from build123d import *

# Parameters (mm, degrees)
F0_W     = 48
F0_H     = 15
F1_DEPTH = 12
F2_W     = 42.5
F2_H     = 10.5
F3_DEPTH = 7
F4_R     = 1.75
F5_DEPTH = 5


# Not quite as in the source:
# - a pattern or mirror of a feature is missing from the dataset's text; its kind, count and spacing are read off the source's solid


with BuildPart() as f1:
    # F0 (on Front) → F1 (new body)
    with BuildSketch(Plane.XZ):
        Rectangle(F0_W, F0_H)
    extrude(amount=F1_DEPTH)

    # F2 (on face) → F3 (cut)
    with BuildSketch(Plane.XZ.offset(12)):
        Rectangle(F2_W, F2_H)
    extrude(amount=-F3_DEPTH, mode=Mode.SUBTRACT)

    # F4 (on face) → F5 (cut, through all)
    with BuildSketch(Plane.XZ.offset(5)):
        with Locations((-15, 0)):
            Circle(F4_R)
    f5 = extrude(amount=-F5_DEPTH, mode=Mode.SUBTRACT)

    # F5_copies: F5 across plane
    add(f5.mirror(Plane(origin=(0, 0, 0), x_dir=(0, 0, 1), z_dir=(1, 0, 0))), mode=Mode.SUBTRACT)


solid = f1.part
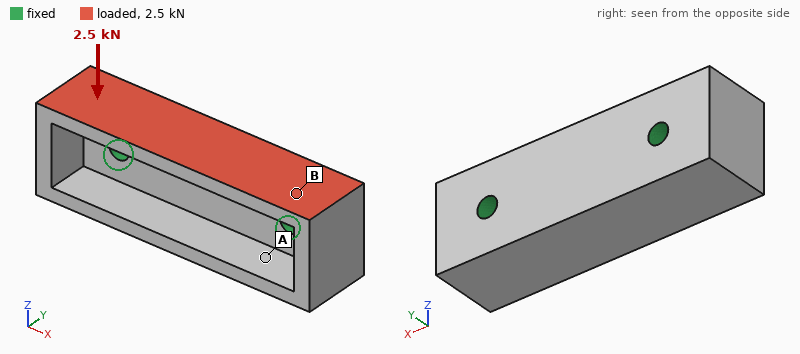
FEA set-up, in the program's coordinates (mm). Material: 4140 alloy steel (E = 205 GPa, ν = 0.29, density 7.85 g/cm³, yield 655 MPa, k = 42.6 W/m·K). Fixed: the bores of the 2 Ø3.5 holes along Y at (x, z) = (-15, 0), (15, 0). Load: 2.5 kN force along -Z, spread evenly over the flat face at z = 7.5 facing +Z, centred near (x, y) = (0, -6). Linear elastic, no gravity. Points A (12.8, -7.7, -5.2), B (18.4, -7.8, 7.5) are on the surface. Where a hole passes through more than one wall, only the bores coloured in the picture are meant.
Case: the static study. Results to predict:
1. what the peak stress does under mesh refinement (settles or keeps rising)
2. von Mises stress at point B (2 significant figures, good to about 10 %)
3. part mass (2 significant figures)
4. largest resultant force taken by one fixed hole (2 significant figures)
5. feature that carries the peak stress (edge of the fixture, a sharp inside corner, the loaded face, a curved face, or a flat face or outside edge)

keeps rising
47 MPa
43 g
1.3 kN
edge of the fixture
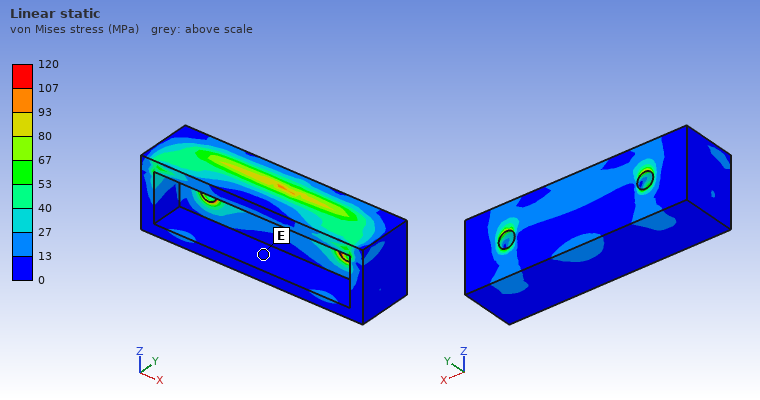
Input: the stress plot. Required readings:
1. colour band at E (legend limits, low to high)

0 to 13 MPa
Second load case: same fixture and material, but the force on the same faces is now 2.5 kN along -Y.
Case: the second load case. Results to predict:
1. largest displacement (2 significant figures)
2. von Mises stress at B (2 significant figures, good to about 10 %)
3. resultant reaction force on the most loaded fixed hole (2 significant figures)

18 µm
27 MPa
1.3 kN
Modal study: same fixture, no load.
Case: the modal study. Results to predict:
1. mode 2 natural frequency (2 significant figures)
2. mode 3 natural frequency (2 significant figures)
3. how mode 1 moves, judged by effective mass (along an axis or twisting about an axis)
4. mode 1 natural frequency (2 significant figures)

22 kHz
24 kHz
along Z
18 kHz
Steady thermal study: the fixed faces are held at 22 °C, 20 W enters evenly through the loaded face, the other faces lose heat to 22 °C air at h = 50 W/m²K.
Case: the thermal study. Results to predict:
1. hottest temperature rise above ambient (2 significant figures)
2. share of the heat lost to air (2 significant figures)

31 K
8.3 %
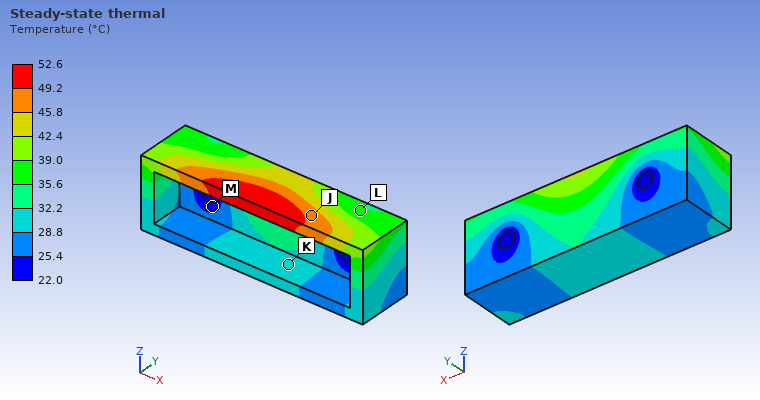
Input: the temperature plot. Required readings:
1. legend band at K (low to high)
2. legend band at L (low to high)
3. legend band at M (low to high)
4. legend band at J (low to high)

28.8 to 32.2 °C
35.6 to 39.0 °C
22.0 to 25.4 °C
45.8 to 49.2 °C
